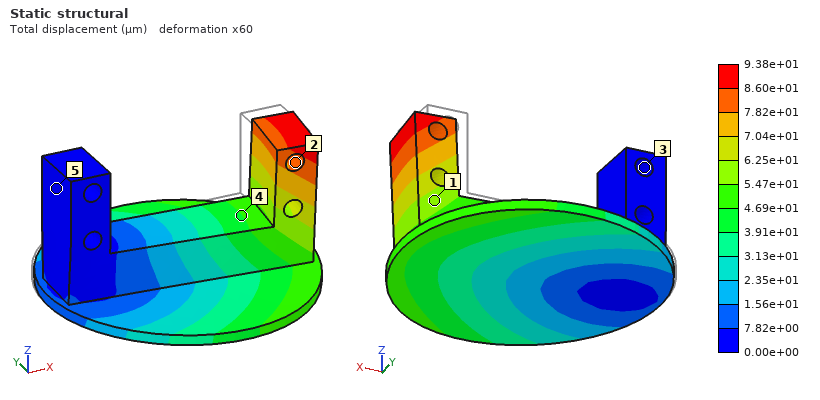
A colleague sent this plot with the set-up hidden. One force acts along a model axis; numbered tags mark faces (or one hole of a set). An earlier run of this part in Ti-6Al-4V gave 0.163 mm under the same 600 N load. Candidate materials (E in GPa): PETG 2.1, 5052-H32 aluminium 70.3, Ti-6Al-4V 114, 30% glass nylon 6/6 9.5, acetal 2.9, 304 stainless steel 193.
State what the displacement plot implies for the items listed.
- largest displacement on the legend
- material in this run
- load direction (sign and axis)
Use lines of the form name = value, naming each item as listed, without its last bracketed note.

largest displacement on the legend = 9.38e+01 µm
material in this run = 304 stainless steel
load direction = -Y
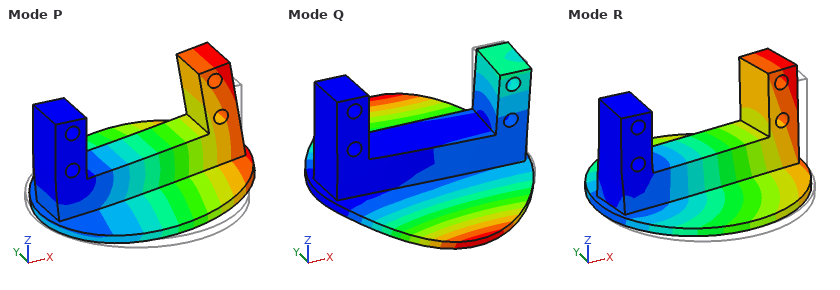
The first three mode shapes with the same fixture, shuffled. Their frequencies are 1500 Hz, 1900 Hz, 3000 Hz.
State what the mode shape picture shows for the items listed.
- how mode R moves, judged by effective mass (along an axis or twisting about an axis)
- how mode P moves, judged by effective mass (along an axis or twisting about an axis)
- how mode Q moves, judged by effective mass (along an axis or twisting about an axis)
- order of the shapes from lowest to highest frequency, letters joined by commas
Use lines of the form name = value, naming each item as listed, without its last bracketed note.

how mode R moves, judged by effective mass = along Y
how mode P moves, judged by effective mass = along Z
how mode Q moves, judged by effective mass = twisting about X
order of the shapes from lowest to highest frequency, letters joined by commas = P, R, Q
